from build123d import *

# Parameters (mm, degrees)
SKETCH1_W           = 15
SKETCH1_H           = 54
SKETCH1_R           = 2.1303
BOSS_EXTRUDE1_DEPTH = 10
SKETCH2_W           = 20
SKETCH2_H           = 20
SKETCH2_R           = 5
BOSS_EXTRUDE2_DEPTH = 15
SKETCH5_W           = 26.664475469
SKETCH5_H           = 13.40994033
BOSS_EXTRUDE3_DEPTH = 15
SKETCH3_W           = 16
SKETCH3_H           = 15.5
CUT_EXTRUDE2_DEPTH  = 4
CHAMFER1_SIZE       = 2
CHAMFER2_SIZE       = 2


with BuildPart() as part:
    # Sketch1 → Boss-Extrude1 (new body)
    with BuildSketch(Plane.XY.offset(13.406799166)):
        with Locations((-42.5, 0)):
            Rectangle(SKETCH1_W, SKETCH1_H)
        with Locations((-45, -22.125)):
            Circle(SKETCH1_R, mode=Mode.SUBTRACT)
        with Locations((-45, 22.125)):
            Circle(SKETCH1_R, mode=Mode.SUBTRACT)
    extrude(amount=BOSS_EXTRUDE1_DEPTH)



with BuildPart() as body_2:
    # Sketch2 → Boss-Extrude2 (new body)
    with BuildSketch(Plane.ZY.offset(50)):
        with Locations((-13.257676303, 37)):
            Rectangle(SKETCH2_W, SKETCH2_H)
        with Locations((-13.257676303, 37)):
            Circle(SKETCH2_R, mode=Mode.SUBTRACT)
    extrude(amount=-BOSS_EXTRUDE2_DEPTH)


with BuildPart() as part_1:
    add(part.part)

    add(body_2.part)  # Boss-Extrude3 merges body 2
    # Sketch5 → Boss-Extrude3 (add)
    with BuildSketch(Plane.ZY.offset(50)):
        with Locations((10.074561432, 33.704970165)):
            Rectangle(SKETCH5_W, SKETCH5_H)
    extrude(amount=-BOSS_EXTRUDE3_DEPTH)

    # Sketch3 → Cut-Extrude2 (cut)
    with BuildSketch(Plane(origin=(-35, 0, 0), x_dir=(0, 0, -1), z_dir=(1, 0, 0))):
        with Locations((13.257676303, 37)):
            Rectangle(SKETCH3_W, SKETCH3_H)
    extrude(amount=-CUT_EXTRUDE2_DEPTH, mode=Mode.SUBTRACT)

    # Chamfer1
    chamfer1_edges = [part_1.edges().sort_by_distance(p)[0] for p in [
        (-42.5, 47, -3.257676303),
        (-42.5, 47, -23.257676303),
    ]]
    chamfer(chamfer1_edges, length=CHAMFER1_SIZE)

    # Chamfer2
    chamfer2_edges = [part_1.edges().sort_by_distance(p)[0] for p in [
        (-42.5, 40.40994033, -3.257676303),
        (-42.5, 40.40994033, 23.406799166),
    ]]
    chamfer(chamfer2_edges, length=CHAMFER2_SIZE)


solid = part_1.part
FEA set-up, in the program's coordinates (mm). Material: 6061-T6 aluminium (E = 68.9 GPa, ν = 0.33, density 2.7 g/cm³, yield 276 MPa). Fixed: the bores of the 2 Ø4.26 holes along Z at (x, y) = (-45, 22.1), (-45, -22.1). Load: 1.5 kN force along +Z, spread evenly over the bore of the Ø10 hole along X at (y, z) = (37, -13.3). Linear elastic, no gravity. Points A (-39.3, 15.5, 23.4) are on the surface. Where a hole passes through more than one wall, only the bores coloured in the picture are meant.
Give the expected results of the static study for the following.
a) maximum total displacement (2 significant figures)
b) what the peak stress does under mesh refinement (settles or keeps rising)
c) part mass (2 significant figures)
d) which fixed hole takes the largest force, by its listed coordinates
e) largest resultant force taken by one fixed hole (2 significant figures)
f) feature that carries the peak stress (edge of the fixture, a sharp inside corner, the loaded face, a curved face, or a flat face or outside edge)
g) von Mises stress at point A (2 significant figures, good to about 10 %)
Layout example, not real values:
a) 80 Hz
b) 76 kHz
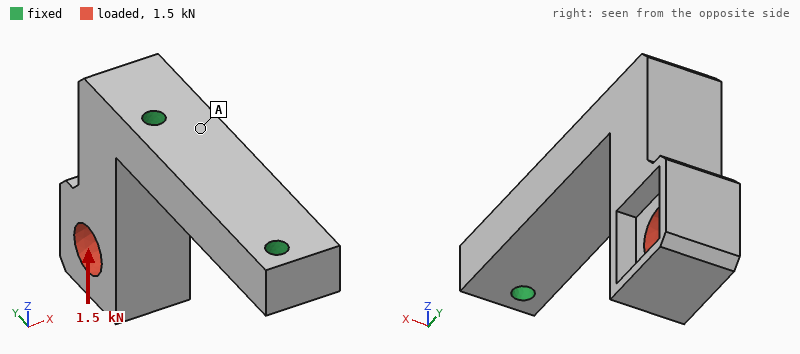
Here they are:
a) 0.11 mm
b) keeps rising
c) 47 g
d) (-45, 22.1)
e) 1.6 kN
f) edge of the fixture
g) 13 MPa
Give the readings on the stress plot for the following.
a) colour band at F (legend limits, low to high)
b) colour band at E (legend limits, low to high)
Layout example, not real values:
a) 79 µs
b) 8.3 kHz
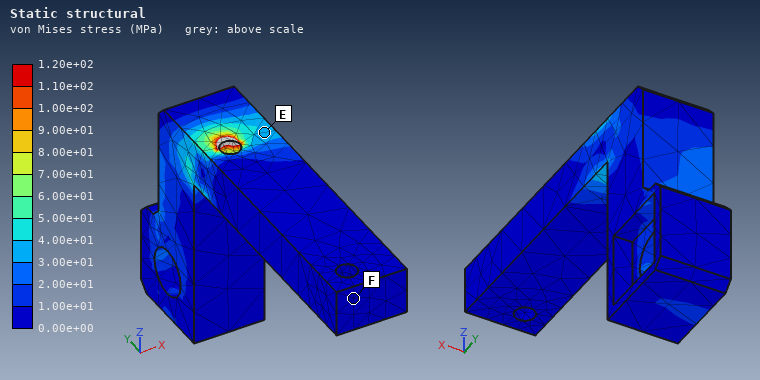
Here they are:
a) 0.00e+00 to 1.00e+01 MPa
b) 3.00e+01 to 4.00e+01 MPa
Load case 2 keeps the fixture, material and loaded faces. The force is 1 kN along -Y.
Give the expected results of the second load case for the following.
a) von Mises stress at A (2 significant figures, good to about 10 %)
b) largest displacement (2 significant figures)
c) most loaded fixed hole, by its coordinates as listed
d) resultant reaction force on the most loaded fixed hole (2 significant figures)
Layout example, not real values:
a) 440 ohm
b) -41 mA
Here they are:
a) 18 MPa
b) 0.24 mm
c) (-45, 22.1)
d) 960 N
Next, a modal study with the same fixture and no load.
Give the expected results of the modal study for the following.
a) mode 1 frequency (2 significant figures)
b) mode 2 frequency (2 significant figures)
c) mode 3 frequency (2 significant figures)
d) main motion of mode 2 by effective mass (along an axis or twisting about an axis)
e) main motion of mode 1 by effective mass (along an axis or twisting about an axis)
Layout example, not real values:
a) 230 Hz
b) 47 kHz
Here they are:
a) 3200 Hz
b) 3500 Hz
c) 10 kHz
d) along X
e) along Y
